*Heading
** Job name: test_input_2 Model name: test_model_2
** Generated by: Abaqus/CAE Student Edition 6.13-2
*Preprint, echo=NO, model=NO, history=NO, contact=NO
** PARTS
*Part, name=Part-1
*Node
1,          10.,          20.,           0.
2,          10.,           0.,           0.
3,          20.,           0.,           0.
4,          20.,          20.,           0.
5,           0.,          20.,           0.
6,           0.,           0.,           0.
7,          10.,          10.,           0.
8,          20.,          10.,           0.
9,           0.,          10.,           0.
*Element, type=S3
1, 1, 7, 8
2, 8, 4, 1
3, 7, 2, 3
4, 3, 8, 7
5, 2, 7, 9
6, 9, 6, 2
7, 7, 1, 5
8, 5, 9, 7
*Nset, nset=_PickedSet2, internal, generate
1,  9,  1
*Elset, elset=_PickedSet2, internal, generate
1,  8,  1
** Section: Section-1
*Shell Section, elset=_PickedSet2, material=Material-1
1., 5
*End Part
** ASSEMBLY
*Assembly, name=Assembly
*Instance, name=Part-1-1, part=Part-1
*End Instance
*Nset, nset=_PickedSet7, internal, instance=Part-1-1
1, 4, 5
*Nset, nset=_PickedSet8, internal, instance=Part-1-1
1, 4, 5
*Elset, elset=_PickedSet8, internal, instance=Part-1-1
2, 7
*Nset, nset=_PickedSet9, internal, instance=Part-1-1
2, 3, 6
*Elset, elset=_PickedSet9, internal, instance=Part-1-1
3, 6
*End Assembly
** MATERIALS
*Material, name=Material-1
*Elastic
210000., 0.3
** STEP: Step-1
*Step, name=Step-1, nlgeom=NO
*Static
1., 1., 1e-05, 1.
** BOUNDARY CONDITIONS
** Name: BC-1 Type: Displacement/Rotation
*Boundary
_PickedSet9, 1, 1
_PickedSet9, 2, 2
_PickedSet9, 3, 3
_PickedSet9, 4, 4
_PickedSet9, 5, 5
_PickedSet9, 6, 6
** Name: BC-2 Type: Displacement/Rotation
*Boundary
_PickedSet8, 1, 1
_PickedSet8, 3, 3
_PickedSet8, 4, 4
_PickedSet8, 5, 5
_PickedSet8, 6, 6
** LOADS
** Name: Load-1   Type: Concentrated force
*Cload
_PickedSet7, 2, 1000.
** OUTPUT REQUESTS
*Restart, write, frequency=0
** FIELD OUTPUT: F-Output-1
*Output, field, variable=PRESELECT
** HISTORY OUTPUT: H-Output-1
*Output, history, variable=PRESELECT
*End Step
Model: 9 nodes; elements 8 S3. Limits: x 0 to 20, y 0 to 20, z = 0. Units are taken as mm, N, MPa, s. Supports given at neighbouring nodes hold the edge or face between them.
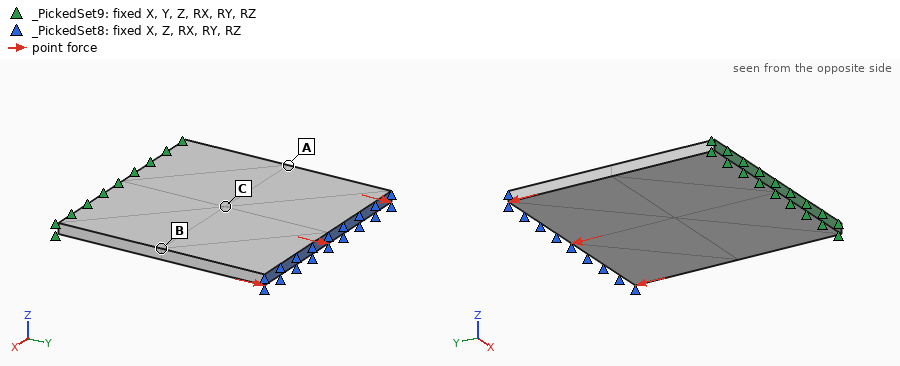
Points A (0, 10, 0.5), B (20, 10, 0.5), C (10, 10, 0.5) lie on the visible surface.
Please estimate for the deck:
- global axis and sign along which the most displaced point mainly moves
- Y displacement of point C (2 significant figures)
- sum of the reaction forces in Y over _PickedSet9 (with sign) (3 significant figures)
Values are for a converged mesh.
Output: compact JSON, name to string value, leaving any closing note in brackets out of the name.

{"global axis and sign along which the most displaced point mainly moves": "+Y", "Y displacement of point C": "0.0067 mm", "sum of the reaction forces in Y over _PickedSet9 (with sign)": "-3000 N"}
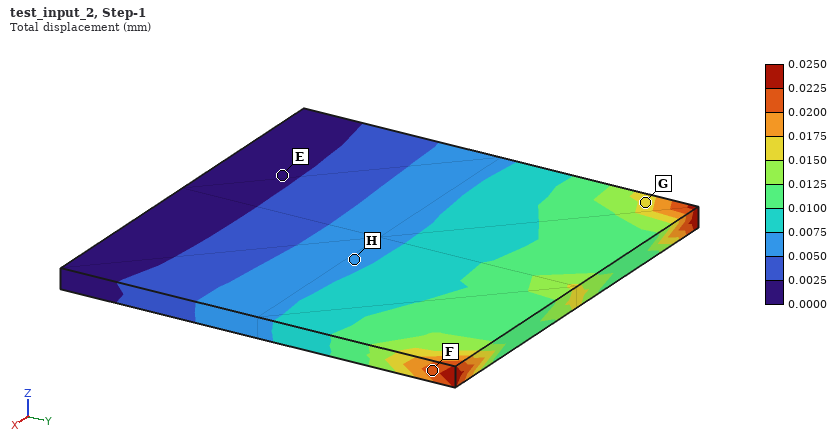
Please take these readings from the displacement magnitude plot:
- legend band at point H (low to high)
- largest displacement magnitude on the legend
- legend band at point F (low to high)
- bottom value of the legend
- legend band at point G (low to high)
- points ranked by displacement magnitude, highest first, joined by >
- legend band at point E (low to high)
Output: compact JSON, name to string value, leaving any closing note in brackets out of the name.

{"legend band at point H": "0.0050 to 0.0075 mm", "largest displacement magnitude on the legend": "0.0250 mm", "legend band at point F": "0.0200 to 0.0225 mm", "bottom value of the legend": "0.0000 mm", "legend band at point G": "0.0150 to 0.0175 mm", "points ranked by displacement magnitude, highest first, joined by >": "F > G > H > E", "legend band at point E": "0.0000 to 0.0025 mm"}
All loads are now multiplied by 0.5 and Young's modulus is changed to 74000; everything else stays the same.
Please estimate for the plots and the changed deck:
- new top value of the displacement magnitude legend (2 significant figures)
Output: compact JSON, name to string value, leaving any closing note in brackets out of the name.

{"new top value of the displacement magnitude legend": "0.035 mm"}
